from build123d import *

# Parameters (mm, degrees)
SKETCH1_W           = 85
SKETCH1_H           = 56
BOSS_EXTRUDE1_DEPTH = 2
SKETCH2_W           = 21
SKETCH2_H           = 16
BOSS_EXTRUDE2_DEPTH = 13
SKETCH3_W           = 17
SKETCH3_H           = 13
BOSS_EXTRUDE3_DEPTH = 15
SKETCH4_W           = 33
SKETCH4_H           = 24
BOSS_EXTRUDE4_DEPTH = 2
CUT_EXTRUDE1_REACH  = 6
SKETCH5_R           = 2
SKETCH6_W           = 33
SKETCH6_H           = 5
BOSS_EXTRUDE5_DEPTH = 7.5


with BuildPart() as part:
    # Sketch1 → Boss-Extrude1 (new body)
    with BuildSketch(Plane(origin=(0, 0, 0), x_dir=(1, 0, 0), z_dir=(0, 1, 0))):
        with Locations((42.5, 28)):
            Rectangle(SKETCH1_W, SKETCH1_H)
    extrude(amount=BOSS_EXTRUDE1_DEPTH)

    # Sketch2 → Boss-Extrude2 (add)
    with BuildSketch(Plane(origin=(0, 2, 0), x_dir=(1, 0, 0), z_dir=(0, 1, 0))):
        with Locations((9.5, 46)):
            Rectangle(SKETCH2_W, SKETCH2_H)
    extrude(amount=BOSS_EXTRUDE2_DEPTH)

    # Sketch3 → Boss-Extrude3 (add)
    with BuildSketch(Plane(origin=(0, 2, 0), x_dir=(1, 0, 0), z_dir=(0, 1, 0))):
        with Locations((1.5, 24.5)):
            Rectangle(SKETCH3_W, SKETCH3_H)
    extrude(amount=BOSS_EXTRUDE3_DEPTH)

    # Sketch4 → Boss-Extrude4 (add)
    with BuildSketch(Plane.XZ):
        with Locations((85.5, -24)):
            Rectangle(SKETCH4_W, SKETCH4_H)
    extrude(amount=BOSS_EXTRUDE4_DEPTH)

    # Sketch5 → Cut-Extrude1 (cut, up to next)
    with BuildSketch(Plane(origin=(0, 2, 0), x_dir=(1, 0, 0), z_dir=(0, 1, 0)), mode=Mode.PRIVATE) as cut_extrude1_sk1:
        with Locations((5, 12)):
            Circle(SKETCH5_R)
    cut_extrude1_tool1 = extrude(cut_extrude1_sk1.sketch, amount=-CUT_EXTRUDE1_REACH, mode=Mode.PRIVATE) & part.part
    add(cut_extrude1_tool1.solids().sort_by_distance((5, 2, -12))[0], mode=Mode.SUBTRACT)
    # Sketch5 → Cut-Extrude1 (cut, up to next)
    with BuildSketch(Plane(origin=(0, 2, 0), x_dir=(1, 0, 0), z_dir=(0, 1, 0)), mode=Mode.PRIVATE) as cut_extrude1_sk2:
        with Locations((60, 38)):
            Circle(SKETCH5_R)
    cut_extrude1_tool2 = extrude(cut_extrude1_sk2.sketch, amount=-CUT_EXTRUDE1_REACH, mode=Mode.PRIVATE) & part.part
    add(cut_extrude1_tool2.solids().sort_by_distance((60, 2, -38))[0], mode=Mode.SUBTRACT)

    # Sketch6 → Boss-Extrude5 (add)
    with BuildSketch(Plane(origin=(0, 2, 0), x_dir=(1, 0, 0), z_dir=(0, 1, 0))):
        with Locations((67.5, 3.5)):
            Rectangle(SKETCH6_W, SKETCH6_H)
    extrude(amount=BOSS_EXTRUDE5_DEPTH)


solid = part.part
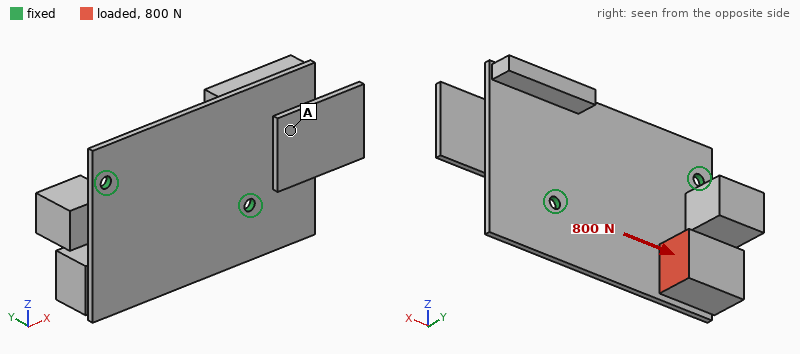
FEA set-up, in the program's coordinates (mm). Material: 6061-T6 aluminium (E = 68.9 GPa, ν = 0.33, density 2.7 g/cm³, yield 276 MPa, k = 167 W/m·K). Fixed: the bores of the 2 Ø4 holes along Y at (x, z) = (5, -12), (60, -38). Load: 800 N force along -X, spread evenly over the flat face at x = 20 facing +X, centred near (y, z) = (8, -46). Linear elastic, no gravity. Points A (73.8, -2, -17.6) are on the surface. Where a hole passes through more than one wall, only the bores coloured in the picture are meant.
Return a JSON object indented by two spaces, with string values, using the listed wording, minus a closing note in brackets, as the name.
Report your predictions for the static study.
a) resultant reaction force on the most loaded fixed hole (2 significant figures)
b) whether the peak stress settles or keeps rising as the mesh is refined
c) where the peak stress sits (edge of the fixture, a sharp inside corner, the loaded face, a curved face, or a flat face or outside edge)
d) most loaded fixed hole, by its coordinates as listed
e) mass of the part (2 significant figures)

{
  "resultant reaction force on the most loaded fixed hole": "610 N",
  "whether the peak stress settles or keeps rising as the mesh is refined": "keeps rising",
  "where the peak stress sits": "edge of the fixture",
  "most loaded fixed hole, by its coordinates as listed": "(60, -38)",
  "mass of the part": "54 g"
}
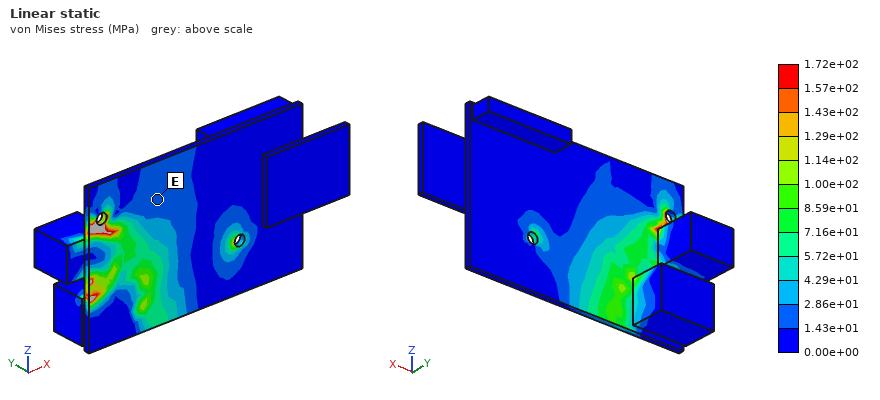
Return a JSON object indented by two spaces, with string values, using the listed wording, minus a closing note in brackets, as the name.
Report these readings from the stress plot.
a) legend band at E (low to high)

{
  "legend band at E": "1.43e+01 to 2.86e+01 MPa"
}
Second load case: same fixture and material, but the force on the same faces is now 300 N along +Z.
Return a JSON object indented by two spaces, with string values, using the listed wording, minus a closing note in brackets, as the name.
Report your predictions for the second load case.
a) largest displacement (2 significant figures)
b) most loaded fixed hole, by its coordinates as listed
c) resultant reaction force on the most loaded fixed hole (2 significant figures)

{
  "largest displacement": "0.48 mm",
  "most loaded fixed hole, by its coordinates as listed": "(5, -12)",
  "resultant reaction force on the most loaded fixed hole": "220 N"
}
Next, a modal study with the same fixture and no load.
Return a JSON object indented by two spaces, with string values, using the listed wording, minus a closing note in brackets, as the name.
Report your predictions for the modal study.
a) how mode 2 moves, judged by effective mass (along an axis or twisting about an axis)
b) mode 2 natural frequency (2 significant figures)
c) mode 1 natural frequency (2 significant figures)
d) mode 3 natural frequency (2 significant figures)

{
  "how mode 2 moves, judged by effective mass": "along Y",
  "mode 2 natural frequency": "790 Hz",
  "mode 1 natural frequency": "610 Hz",
  "mode 3 natural frequency": "1500 Hz"
}
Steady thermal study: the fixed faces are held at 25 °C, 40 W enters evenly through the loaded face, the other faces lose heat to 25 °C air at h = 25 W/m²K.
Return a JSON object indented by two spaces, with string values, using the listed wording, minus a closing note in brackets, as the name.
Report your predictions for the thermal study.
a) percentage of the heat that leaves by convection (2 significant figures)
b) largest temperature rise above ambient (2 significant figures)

{
  "percentage of the heat that leaves by convection": "21 %",
  "largest temperature rise above ambient": "80 K"
}
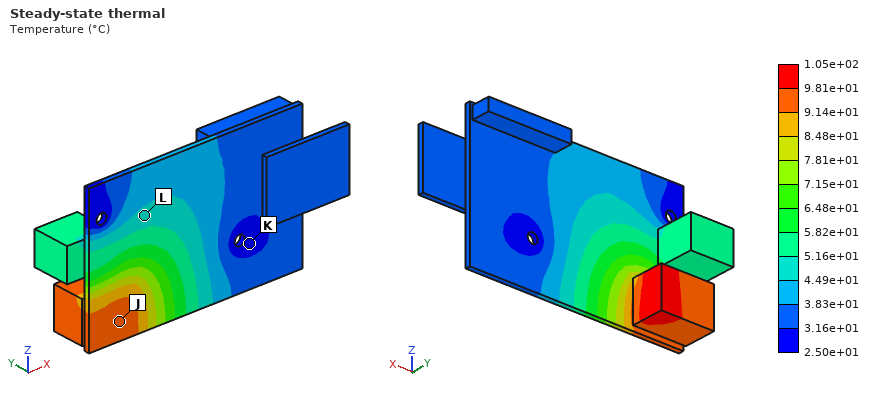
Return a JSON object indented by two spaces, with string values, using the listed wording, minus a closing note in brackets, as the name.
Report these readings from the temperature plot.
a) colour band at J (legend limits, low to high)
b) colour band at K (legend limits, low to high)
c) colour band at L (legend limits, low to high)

{
  "colour band at J": "9.14e+01 to 9.81e+01 °C",
  "colour band at K": "2.50e+01 to 3.16e+01 °C",
  "colour band at L": "4.49e+01 to 5.16e+01 °C"
}
